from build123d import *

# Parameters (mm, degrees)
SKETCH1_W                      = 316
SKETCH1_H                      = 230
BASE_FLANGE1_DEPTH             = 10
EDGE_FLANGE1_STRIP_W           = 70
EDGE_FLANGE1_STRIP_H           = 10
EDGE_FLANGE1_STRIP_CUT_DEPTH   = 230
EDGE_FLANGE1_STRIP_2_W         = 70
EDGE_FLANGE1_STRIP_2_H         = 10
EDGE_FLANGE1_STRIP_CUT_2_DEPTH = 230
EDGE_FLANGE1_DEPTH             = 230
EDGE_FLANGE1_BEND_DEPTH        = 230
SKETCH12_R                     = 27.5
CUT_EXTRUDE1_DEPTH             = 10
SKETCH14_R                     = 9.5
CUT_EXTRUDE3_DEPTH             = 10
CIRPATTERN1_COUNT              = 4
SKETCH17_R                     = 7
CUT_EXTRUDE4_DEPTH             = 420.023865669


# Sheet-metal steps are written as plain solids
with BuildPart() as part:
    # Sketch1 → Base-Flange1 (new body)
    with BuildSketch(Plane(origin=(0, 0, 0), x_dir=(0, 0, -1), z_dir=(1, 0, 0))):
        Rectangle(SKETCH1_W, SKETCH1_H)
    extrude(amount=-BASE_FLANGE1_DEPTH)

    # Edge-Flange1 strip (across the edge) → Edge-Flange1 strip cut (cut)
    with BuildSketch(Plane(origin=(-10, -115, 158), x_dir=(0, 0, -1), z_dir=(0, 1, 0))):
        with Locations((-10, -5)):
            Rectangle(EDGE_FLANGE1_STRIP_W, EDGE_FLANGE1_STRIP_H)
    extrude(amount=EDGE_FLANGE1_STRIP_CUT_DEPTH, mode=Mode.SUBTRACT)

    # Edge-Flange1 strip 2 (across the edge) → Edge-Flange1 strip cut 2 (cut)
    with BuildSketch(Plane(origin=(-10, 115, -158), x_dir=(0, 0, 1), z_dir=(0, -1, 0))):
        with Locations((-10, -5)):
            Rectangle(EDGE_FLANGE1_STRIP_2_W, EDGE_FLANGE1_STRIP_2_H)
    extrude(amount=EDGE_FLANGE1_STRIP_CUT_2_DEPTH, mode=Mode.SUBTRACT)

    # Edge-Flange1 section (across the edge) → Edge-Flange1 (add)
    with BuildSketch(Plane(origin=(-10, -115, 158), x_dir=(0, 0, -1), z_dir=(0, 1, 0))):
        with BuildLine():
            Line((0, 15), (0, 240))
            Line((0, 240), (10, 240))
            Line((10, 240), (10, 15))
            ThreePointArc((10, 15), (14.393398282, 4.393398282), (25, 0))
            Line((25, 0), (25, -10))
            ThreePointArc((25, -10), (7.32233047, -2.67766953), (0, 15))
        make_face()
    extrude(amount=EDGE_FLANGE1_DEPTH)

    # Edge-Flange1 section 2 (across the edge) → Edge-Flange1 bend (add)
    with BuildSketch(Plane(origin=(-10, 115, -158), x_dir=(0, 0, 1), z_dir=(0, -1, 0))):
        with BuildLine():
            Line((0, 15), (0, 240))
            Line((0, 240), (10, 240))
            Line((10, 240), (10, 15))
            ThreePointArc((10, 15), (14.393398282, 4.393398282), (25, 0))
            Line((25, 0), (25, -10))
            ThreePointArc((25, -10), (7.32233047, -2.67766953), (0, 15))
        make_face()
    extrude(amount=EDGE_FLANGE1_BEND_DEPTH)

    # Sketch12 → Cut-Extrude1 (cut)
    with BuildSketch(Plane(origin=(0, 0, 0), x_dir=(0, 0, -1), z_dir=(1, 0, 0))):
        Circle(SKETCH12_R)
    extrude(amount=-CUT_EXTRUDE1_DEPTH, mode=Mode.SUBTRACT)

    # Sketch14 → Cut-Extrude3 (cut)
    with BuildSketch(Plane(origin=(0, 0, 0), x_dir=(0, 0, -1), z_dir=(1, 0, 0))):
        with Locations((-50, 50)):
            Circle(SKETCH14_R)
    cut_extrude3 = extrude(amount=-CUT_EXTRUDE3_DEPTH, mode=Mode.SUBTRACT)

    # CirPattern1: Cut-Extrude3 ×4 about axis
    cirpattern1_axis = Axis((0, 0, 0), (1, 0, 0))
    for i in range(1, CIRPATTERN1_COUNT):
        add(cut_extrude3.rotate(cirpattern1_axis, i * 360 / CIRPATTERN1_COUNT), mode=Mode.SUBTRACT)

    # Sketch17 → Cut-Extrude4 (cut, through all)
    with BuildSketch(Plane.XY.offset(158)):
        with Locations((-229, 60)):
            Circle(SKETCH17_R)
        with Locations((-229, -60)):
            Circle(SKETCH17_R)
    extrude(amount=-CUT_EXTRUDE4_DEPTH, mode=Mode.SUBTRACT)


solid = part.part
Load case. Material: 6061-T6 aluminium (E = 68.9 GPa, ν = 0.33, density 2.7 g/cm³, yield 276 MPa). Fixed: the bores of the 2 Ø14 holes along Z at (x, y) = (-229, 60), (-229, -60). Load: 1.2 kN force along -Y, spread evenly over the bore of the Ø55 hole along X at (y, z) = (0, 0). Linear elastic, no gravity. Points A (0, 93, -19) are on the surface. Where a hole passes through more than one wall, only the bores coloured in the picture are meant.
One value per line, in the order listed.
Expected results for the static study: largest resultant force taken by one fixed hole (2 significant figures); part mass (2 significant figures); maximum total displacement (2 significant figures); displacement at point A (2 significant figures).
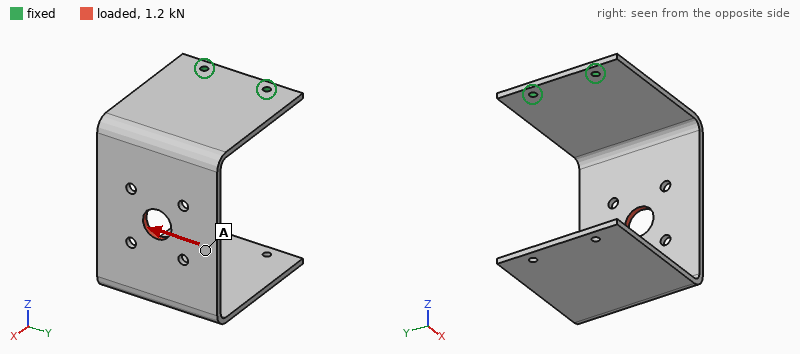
2.5 kN
4.7 kg
5.4 mm
2.8 mm
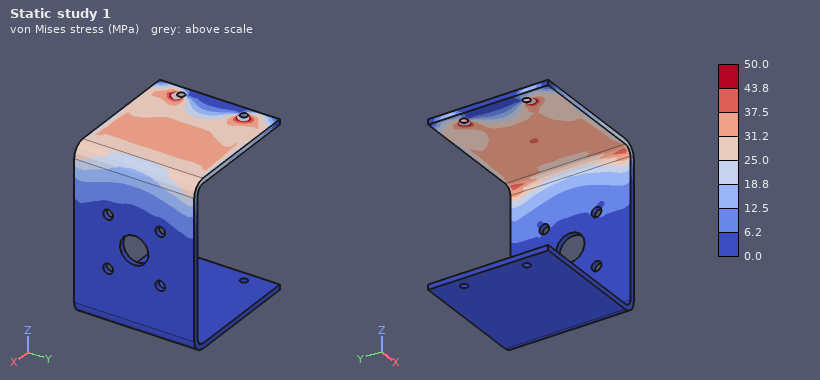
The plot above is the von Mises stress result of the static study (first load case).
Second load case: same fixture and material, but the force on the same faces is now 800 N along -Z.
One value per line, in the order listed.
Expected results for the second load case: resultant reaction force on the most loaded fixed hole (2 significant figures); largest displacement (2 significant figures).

400 N
5.2 mm
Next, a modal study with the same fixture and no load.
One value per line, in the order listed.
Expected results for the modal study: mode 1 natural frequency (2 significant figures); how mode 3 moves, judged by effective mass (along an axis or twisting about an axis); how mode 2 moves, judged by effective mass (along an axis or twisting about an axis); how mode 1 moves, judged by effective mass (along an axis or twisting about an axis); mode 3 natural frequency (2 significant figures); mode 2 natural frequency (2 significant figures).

22 Hz
along Z
along Y
along X
55 Hz
35 Hz
